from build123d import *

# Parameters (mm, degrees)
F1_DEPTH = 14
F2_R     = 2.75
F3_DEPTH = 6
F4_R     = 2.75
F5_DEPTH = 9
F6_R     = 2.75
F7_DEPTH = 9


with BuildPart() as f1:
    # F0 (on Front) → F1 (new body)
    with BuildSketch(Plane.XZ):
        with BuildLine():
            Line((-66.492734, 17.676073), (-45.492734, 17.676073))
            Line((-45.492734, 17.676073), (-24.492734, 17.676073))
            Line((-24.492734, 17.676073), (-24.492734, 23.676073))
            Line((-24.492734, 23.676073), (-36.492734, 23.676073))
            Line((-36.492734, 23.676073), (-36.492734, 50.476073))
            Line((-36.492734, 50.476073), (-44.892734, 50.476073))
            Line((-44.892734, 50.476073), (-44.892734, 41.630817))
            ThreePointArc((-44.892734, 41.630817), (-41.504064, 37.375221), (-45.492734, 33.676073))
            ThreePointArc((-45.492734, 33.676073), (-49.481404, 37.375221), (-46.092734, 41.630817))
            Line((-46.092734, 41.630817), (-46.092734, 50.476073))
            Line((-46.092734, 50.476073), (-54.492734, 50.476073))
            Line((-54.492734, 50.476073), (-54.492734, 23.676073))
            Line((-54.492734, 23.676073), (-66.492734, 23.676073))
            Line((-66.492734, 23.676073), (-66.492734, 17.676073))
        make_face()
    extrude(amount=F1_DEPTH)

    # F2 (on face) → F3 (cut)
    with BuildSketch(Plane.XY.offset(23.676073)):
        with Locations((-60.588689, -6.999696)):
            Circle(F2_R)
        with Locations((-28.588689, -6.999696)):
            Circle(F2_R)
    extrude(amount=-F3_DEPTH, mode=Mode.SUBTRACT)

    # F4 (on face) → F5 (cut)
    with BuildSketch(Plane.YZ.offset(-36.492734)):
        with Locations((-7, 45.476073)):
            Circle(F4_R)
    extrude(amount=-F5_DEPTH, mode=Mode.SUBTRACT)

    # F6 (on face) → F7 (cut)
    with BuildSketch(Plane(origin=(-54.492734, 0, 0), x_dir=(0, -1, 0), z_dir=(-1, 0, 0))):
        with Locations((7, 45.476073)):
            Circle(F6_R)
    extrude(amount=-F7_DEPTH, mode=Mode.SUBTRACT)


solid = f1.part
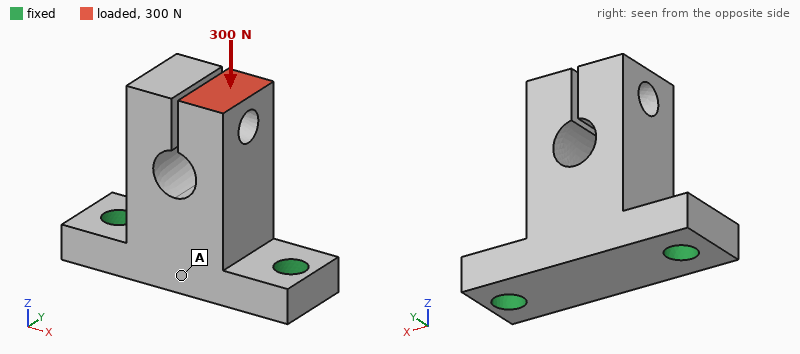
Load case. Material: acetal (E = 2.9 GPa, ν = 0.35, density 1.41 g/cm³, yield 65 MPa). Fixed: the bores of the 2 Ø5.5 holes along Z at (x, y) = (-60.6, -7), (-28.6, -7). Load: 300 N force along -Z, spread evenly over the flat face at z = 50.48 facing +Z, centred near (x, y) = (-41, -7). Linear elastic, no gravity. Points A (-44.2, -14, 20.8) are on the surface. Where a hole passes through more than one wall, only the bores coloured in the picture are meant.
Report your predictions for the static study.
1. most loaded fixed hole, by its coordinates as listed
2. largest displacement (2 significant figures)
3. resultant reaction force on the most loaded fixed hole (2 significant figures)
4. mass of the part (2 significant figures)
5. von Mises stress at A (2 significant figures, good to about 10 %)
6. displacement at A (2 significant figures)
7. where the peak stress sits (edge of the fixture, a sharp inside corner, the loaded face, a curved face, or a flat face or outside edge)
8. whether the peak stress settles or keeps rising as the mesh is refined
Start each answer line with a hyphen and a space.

- (-28.6, -7)
- 0.13 mm
- 210 N
- 12 g
- 1.6 MPa
- 0.032 mm
- edge of the fixture
- keeps rising
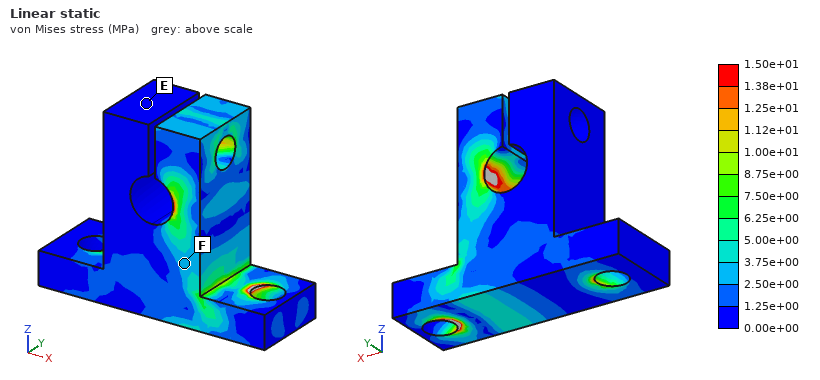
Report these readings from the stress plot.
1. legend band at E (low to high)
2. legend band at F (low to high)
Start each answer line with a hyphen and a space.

- 0.00e+00 to 1.25e+00 MPa
- 2.50e+00 to 3.75e+00 MPa
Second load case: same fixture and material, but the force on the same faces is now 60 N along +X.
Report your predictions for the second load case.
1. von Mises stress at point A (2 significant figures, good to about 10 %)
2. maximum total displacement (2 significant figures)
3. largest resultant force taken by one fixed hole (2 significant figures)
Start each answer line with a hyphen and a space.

- 1.4 MPa
- 0.30 mm
- 86 N
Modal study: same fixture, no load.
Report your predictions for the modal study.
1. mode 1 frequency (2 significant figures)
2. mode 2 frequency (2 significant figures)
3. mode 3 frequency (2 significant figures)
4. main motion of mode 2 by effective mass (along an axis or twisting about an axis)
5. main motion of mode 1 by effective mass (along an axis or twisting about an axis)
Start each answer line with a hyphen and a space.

- 1500 Hz
- 2400 Hz
- 2900 Hz
- along X
- along Y
